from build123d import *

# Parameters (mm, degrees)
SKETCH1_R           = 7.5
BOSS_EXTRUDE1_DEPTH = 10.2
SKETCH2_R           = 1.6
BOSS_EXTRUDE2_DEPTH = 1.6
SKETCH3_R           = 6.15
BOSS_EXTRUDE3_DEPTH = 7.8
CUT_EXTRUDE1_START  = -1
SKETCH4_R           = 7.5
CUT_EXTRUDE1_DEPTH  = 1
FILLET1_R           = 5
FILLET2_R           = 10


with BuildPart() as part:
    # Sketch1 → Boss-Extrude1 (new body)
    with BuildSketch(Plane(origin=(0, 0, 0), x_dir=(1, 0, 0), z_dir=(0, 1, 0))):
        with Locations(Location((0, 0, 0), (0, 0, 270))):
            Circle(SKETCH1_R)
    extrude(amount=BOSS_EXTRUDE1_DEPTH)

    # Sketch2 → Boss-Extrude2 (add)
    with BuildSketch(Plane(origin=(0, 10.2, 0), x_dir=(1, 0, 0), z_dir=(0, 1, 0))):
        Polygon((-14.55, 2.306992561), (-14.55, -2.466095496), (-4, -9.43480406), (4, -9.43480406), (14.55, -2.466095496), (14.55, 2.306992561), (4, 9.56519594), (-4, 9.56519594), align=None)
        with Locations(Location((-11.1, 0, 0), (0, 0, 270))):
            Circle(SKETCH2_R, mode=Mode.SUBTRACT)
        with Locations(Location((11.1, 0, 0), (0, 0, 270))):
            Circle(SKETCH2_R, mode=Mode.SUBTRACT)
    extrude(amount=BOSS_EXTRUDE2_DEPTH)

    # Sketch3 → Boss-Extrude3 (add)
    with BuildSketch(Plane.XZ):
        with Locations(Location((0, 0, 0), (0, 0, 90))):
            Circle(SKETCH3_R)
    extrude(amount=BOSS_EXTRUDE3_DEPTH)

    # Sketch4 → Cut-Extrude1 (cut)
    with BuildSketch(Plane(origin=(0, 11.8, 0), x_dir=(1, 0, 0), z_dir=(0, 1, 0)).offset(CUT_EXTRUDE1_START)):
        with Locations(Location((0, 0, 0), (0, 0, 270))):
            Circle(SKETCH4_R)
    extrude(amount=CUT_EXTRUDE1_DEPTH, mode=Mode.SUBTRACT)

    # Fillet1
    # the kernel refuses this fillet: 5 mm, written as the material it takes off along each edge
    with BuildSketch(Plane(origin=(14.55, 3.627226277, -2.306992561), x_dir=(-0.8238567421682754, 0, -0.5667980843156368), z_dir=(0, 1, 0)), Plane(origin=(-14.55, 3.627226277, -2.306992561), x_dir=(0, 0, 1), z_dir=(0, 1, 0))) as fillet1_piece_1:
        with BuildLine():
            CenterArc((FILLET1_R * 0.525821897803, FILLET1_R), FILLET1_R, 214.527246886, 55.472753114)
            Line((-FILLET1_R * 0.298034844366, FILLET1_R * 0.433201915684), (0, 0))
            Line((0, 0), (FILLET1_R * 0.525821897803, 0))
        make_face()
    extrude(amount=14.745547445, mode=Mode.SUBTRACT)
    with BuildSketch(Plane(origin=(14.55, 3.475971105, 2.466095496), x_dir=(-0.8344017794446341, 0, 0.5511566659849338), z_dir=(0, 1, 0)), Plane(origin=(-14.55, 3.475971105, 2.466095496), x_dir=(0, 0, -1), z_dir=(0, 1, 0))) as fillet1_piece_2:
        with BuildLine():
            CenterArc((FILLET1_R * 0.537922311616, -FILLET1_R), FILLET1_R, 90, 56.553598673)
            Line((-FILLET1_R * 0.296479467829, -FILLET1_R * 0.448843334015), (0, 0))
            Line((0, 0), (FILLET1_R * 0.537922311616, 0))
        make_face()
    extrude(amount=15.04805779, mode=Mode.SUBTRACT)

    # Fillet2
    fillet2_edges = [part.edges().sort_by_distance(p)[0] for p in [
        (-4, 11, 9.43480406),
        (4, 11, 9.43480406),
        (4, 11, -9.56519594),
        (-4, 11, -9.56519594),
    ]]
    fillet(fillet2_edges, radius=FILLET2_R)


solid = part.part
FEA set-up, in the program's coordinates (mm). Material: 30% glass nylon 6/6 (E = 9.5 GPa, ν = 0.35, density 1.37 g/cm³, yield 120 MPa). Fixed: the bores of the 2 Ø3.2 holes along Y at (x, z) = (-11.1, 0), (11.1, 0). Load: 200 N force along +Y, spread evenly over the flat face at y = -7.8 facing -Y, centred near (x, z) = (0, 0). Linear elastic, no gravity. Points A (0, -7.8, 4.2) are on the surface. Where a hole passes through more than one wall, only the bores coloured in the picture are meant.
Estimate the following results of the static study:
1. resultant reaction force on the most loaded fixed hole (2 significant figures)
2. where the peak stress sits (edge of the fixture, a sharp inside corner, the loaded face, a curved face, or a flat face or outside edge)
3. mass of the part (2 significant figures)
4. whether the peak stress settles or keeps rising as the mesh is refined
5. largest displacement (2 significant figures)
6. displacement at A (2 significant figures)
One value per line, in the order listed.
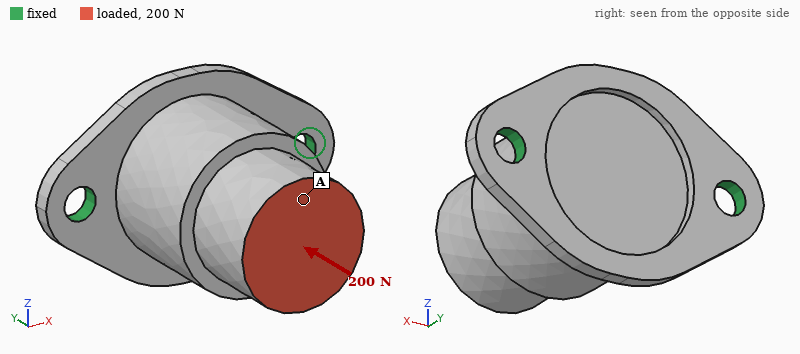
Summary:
130 N
edge of the fixture
4.3 g
keeps rising
29 µm
29 µm
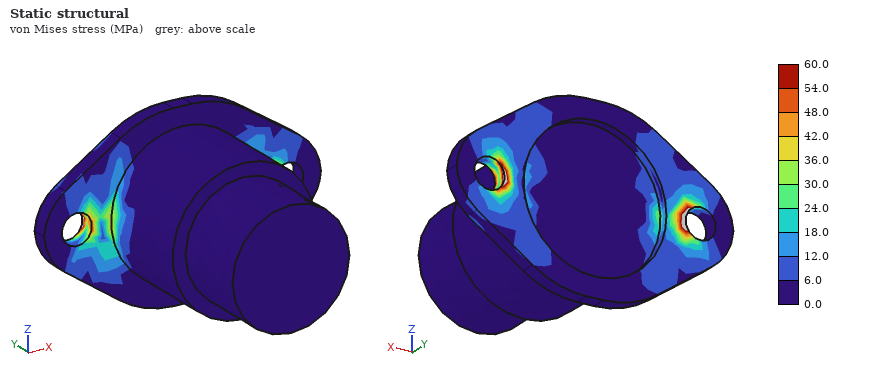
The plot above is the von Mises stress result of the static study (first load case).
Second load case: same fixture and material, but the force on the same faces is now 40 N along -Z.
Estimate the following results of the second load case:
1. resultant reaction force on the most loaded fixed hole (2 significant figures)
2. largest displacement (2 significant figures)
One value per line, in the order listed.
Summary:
20 N
0.40 mm
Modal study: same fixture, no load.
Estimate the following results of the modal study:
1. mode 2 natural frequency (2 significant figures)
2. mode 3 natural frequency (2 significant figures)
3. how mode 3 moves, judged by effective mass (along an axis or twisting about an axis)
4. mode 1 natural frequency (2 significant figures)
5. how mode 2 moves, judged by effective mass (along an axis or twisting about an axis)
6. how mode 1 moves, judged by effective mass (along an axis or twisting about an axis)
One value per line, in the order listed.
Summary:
5200 Hz
6700 Hz
along Y
1400 Hz
along X
along Z
